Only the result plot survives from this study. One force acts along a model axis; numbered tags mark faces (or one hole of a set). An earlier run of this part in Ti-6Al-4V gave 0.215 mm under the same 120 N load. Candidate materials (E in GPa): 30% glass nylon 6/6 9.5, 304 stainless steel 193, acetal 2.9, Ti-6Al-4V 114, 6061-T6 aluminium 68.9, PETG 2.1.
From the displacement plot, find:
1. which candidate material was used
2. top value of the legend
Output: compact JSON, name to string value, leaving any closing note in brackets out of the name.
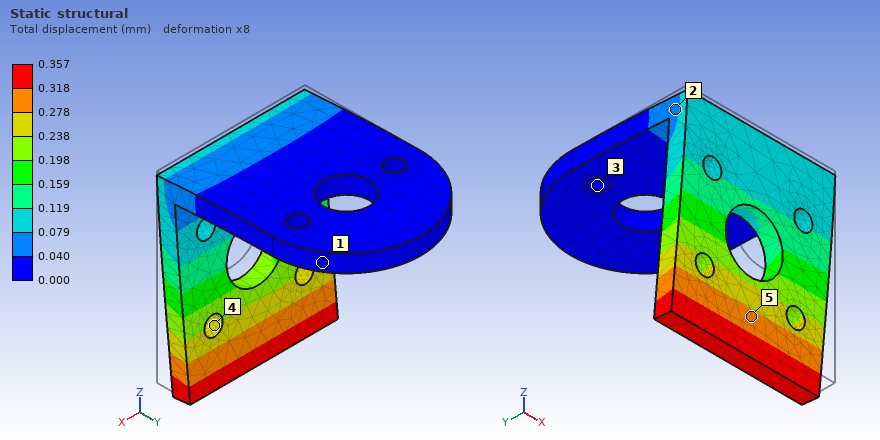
{"which candidate material was used": "6061-T6 aluminium", "top value of the legend": "0.357 mm"}
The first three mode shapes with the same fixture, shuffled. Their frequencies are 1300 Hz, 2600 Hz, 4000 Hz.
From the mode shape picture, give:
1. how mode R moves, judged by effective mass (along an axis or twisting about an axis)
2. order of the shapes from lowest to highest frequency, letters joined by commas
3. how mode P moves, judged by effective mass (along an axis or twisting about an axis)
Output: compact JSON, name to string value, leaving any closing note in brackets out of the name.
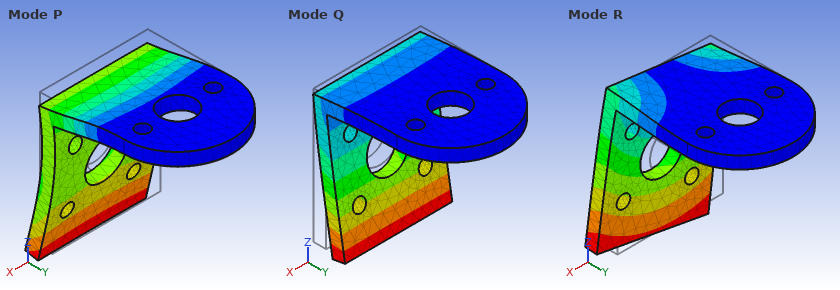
{"how mode R moves, judged by effective mass": "along X", "order of the shapes from lowest to highest frequency, letters joined by commas": "Q, R, P", "how mode P moves, judged by effective mass": "along Z"}
